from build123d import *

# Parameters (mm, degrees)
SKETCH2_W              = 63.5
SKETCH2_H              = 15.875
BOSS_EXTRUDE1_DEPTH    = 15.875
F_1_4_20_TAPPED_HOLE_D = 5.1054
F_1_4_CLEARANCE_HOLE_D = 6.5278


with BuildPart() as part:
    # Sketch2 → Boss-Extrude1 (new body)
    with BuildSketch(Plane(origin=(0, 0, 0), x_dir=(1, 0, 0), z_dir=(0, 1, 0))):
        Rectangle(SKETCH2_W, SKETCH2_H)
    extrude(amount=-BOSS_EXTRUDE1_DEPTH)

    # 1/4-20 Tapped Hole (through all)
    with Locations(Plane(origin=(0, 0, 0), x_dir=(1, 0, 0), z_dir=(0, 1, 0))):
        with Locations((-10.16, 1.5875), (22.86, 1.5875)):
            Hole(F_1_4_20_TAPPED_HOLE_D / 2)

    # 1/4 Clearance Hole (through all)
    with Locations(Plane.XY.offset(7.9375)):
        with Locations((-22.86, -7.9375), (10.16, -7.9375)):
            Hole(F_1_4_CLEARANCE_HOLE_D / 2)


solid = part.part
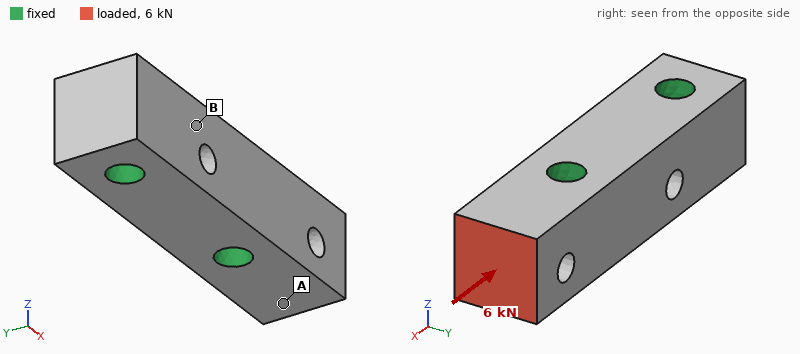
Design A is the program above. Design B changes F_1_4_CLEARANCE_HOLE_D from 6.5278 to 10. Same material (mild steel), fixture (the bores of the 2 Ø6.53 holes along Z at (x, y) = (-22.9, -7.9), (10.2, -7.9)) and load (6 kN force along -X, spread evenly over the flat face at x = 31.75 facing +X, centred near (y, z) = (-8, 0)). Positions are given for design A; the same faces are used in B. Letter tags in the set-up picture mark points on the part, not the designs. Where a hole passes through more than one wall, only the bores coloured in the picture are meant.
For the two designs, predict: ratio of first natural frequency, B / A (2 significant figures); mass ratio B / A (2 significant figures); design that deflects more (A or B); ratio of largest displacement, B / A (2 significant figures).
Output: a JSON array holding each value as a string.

["1.2", "0.90", "A", "0.91"]
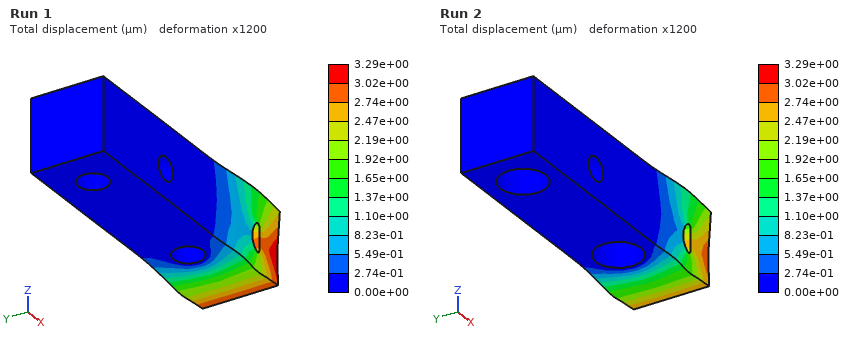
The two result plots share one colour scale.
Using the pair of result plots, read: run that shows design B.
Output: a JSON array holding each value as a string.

["Run 2"]
